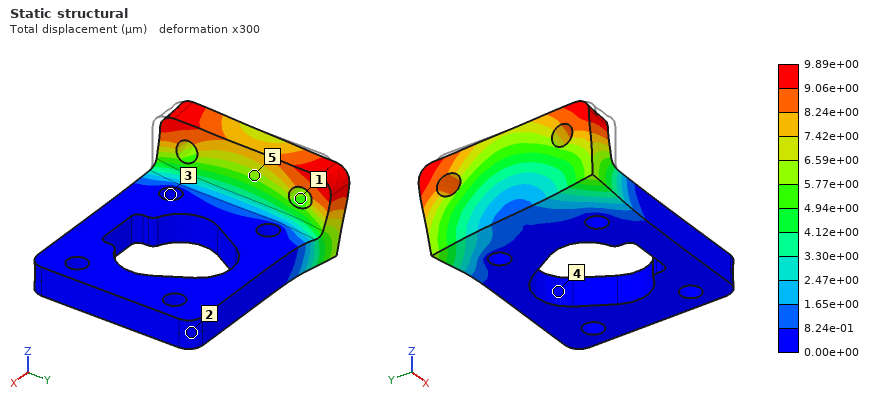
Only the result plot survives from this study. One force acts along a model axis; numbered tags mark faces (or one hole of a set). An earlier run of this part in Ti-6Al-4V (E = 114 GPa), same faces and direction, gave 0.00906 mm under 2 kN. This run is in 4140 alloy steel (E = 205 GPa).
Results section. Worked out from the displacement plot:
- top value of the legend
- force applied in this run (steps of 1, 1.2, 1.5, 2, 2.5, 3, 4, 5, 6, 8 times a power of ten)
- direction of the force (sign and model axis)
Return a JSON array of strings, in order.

["9.89e+00 µm", "4 kN", "+Y"]
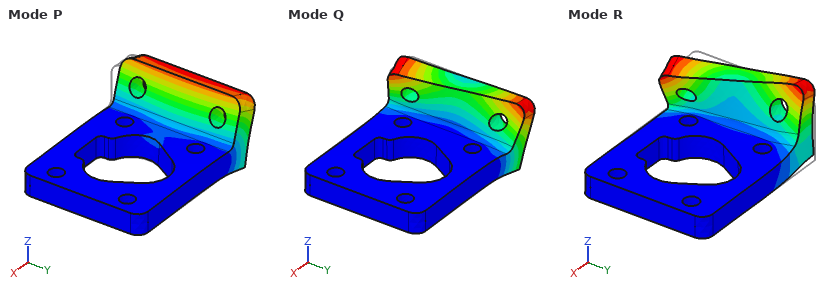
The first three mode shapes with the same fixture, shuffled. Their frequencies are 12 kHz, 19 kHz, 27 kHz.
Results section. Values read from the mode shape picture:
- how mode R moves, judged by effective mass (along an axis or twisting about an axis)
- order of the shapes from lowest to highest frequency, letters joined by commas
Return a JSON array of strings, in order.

["along Y", "P, Q, R"]
